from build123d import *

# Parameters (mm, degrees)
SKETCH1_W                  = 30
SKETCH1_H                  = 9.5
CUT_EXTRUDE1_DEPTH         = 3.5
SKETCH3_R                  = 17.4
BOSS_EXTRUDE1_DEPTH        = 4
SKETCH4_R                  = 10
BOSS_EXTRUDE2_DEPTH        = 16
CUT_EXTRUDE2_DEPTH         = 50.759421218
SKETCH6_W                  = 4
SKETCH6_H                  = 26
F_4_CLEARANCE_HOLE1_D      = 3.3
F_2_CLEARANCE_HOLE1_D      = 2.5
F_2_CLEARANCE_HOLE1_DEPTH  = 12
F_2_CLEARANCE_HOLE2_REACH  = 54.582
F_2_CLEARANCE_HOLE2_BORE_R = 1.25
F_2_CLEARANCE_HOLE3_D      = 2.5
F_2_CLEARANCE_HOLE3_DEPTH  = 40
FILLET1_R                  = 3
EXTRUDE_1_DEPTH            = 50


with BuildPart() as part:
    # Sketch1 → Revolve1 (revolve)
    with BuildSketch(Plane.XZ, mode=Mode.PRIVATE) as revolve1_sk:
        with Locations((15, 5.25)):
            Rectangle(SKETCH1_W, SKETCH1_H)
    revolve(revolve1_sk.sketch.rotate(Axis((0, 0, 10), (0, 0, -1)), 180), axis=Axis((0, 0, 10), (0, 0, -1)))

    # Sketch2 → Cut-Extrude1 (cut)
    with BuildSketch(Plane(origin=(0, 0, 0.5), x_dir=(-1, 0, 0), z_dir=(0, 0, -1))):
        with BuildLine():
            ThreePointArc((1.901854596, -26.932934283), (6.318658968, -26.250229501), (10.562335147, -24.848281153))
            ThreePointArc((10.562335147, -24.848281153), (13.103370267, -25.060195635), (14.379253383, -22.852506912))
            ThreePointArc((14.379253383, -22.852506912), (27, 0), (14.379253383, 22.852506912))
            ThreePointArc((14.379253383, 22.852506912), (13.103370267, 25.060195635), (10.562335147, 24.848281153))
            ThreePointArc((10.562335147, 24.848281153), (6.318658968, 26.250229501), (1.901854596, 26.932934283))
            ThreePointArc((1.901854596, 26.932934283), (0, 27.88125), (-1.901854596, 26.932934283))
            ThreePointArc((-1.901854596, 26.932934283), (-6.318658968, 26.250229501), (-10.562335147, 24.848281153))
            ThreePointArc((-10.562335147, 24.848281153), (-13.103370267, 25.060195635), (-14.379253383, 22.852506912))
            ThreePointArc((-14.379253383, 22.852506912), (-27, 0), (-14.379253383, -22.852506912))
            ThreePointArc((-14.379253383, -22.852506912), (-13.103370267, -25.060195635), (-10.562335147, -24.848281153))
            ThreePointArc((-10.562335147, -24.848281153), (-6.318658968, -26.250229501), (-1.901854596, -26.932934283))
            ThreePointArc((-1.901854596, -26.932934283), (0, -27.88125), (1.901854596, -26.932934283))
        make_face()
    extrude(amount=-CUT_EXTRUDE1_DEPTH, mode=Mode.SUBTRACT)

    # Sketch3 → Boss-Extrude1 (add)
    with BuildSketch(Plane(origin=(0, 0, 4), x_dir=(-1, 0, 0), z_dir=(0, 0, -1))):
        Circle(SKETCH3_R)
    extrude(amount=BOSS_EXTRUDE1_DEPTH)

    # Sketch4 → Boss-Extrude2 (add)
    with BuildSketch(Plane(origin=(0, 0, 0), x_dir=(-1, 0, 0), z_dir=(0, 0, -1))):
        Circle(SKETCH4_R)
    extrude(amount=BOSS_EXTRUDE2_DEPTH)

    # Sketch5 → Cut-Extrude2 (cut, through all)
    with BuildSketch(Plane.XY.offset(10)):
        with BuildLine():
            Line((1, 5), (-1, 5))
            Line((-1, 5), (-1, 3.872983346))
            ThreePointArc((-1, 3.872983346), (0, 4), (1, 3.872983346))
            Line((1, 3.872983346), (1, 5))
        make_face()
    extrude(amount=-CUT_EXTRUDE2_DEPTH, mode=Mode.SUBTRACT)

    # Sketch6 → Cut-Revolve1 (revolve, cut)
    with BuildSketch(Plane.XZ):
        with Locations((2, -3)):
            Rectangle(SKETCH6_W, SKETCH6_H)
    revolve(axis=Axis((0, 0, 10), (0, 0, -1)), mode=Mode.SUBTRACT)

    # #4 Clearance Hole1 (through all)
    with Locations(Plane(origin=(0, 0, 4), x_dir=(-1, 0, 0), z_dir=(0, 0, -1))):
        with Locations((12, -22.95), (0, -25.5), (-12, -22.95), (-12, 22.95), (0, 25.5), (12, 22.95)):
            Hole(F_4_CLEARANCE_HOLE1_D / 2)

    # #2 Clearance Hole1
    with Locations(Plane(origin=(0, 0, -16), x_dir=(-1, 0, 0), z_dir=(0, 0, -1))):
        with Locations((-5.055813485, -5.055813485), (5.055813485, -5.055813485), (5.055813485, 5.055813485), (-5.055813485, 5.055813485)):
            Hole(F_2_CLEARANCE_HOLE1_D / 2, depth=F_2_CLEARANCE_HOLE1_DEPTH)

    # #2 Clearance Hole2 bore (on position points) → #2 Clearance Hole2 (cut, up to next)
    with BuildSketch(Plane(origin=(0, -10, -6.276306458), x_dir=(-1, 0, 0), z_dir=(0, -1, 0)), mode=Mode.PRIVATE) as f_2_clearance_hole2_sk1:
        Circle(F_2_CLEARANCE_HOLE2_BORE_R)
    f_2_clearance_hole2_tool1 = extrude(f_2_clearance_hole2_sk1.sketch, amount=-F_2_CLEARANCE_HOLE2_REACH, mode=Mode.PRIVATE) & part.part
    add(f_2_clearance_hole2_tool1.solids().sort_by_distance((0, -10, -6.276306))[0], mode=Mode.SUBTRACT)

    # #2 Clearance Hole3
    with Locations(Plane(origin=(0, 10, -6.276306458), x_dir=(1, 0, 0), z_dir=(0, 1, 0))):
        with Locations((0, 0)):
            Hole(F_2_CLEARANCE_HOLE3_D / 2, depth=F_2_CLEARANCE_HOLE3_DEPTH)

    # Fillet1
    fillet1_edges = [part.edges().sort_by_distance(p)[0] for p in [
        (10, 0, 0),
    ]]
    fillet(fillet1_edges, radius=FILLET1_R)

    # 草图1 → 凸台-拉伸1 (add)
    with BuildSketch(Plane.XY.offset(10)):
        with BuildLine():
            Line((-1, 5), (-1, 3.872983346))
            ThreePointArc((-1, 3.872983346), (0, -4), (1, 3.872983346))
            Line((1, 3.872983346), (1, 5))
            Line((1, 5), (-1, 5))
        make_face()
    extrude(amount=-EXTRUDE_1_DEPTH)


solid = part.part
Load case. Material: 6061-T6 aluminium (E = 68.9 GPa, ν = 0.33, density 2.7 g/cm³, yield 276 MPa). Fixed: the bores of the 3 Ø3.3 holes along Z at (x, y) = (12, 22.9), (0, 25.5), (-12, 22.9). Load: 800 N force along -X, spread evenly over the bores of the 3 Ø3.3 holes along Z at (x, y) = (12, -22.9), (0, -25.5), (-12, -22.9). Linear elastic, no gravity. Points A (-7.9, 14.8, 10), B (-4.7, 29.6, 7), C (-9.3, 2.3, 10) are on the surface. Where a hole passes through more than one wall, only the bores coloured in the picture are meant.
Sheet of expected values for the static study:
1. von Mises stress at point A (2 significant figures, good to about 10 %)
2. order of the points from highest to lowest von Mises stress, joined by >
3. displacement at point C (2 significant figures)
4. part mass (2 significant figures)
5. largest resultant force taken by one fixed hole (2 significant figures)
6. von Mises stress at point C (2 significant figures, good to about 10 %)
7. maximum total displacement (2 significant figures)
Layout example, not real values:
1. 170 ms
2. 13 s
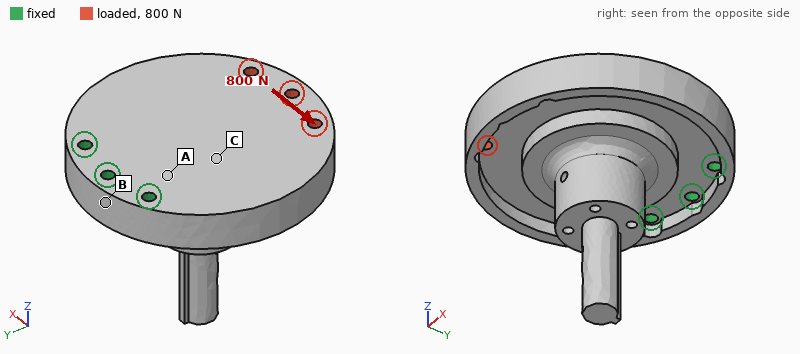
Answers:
1. 16 MPa
2. A > C > B
3. 9.1 µm
4. 77 g
5. 1.5 kN
6. 8.3 MPa
7. 23 µm
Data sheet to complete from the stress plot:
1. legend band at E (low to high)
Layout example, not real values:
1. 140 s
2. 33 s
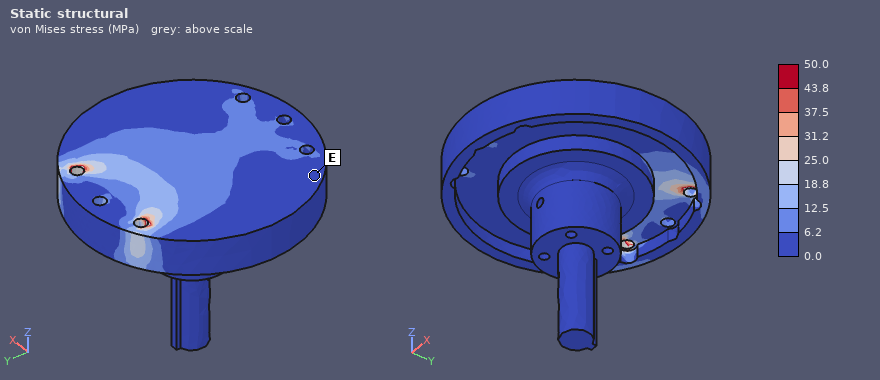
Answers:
1. 0.0 to 6.2 MPa
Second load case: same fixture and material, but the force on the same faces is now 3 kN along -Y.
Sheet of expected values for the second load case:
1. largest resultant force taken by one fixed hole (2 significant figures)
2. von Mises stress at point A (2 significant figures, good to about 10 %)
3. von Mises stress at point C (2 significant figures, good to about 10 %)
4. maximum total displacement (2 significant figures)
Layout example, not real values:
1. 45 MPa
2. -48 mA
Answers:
1. 1.1 kN
2. 14 MPa
3. 14 MPa
4. 22 µm
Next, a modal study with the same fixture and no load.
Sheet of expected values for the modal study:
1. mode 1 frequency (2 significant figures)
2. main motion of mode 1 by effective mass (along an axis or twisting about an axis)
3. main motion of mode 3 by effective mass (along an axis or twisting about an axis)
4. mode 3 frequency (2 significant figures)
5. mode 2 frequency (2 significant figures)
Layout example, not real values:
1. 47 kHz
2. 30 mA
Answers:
1. 1600 Hz
2. along Z
3. along X
4. 6200 Hz
5. 4500 Hz
